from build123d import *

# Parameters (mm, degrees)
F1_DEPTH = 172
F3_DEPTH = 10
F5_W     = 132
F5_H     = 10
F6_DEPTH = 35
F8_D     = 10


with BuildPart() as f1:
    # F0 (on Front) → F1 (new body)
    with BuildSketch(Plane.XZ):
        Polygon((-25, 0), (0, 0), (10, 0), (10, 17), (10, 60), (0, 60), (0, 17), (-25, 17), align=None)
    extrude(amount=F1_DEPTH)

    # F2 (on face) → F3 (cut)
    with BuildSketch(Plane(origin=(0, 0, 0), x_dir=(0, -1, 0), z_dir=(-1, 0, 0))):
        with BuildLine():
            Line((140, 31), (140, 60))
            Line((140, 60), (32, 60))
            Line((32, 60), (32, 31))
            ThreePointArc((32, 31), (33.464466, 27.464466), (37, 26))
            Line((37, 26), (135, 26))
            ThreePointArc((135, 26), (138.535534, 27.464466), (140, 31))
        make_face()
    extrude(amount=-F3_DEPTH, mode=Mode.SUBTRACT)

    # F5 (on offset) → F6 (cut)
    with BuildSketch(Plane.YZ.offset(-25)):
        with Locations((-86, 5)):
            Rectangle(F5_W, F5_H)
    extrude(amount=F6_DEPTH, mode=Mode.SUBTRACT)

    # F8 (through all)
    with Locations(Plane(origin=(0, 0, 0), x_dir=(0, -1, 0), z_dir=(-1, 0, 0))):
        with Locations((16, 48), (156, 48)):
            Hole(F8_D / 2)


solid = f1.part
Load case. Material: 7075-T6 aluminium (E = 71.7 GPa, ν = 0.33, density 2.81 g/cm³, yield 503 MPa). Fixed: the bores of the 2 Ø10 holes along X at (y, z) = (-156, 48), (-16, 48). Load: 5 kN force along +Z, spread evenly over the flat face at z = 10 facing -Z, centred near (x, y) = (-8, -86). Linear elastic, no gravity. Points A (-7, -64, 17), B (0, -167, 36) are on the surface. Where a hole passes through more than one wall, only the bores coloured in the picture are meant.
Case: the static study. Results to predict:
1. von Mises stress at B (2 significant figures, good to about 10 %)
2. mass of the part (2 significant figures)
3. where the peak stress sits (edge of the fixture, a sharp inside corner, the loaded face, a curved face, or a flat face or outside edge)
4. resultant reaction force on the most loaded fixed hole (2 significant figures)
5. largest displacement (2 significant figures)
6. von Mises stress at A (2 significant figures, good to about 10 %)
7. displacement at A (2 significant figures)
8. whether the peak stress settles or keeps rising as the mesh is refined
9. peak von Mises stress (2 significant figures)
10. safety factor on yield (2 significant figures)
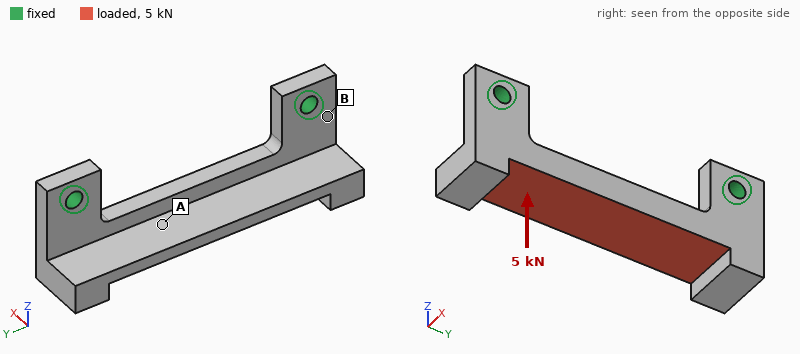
44 MPa
260 g
a curved face
3.1 kN
0.38 mm
18 MPa
0.18 mm
settles
190 MPa
2.6
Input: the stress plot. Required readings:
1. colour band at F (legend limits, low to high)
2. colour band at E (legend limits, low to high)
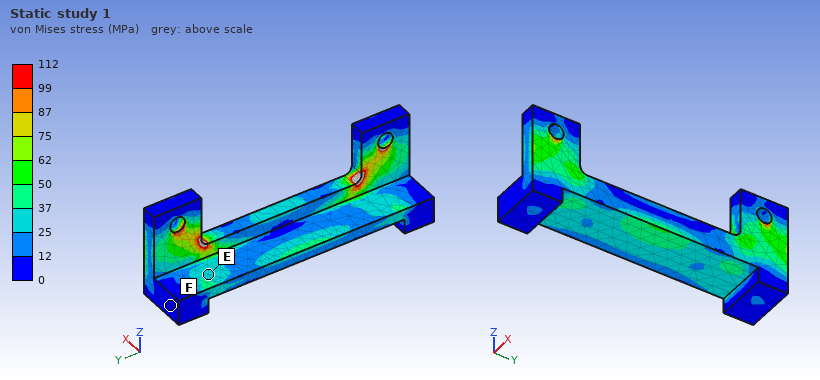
0 to 12 MPa
25 to 37 MPa
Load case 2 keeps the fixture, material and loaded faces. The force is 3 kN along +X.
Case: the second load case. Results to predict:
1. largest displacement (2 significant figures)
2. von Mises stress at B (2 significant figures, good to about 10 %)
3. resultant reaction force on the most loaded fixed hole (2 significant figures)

0.26 mm
58 MPa
1.5 kN
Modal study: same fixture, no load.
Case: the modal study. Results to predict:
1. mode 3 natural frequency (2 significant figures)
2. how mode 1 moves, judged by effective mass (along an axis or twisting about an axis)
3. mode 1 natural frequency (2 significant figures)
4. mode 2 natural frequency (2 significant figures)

3400 Hz
along X
1600 Hz
2300 Hz
